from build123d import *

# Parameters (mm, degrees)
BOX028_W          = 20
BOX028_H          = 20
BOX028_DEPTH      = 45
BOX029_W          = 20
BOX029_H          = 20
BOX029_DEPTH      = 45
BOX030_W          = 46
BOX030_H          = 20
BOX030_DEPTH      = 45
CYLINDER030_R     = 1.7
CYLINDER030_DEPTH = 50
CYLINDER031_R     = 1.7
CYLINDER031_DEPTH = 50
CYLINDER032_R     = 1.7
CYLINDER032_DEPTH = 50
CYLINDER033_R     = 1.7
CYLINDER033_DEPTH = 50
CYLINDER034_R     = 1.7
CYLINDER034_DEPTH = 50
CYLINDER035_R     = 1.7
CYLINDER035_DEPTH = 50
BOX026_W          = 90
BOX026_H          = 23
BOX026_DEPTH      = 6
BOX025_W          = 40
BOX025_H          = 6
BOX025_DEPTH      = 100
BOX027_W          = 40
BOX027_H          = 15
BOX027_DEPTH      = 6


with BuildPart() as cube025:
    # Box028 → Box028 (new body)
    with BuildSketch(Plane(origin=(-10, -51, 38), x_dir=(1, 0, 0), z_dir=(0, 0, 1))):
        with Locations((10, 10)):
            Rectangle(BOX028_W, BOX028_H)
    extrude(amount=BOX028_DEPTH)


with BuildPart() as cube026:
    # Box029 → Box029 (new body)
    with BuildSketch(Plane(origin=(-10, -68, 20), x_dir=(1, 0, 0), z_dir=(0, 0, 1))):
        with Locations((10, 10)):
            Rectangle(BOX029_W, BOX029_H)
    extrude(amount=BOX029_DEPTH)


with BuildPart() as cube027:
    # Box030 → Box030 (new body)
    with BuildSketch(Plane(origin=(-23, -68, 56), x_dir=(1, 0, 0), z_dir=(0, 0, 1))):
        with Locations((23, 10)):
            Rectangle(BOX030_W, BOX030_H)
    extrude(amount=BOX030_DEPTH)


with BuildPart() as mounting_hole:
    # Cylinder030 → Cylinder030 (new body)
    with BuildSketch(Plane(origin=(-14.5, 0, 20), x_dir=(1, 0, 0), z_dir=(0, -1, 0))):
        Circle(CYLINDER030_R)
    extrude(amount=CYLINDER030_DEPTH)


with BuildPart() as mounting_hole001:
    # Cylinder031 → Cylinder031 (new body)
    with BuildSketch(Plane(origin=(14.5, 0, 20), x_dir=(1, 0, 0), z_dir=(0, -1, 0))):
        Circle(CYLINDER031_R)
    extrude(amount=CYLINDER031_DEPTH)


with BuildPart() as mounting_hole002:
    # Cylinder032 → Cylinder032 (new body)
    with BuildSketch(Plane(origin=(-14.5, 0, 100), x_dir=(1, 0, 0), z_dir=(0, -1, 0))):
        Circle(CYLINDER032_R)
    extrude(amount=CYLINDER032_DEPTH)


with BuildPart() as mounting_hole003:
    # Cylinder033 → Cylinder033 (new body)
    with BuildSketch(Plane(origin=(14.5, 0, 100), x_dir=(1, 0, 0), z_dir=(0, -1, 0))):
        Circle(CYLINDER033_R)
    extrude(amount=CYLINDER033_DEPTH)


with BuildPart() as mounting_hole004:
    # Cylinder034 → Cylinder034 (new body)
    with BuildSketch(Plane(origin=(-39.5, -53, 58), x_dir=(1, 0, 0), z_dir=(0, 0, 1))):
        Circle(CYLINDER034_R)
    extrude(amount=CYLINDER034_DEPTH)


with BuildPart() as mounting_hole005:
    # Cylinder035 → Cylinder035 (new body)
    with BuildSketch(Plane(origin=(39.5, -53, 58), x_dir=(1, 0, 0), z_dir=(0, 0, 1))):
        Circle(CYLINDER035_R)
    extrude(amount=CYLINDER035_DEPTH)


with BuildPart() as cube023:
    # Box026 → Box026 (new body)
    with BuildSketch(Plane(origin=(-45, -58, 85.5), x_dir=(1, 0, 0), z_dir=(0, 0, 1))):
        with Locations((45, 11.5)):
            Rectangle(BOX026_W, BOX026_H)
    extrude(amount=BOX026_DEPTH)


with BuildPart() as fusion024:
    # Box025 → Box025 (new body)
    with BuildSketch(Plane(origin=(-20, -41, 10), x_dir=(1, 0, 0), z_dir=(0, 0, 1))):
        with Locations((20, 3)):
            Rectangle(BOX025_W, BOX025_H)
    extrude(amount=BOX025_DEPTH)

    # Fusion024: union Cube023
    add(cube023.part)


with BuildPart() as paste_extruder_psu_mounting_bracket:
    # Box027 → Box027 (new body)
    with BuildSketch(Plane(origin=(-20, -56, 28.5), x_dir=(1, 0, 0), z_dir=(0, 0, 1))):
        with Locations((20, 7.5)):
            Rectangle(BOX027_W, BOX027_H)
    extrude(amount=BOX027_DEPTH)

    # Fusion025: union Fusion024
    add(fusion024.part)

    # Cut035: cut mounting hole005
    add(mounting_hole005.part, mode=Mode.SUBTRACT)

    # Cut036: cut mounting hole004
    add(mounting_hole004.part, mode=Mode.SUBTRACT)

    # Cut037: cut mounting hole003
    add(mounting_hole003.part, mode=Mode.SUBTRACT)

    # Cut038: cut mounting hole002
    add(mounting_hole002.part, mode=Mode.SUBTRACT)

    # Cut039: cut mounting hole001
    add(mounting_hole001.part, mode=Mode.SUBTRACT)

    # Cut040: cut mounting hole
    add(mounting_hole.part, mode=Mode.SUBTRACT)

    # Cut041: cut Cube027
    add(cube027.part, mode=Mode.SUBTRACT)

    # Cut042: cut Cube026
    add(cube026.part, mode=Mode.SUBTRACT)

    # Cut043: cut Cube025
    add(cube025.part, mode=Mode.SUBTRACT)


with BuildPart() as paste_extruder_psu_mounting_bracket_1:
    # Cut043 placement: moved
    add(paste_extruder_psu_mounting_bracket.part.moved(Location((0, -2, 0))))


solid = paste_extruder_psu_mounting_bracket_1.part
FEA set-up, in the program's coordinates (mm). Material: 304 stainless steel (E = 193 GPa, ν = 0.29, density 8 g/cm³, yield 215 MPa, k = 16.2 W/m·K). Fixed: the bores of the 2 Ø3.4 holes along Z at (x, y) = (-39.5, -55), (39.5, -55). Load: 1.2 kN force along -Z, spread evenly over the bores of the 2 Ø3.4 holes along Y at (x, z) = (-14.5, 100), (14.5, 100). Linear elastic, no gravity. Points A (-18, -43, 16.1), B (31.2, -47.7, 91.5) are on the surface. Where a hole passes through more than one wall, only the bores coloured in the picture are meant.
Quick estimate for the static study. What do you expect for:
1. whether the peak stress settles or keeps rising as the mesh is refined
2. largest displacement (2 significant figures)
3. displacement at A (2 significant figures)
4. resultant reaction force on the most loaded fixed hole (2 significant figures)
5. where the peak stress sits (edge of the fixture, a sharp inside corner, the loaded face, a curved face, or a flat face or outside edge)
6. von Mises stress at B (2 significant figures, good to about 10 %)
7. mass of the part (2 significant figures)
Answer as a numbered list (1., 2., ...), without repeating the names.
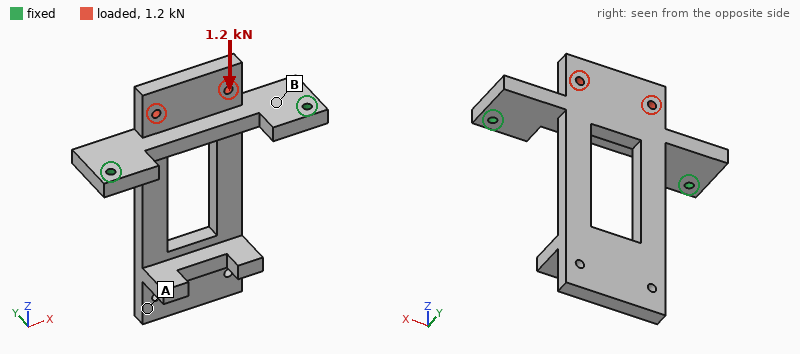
1. keeps rising
2. 0.15 mm
3. 0.13 mm
4. 600 N
5. edge of the fixture
6. 40 MPa
7. 230 g
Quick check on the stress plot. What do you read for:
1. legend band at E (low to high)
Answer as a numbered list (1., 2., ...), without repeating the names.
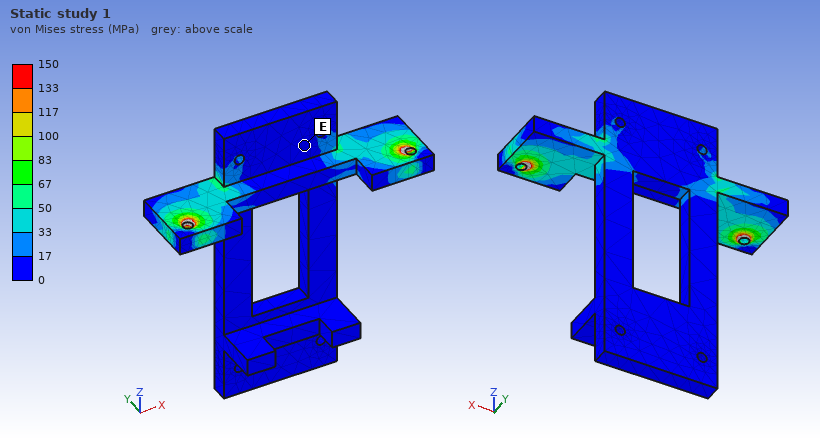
1. 0 to 17 MPa
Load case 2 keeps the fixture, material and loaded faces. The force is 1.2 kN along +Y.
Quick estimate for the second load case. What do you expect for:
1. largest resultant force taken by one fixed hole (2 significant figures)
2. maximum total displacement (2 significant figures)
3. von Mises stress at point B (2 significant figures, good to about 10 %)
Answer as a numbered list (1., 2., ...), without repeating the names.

1. 1.0 kN
2. 0.22 mm
3. 64 MPa
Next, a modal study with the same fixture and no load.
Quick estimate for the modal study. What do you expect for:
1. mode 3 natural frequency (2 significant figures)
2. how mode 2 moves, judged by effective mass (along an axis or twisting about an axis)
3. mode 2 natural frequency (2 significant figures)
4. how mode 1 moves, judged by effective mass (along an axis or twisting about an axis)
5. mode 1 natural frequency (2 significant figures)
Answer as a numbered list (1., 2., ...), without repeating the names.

1. 1900 Hz
2. along X
3. 1300 Hz
4. along Y
5. 400 Hz
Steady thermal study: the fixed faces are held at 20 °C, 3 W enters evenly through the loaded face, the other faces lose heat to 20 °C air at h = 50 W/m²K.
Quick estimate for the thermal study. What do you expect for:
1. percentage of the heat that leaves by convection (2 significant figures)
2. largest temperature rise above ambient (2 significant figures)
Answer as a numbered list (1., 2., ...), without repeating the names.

1. 79 %
2. 16 K
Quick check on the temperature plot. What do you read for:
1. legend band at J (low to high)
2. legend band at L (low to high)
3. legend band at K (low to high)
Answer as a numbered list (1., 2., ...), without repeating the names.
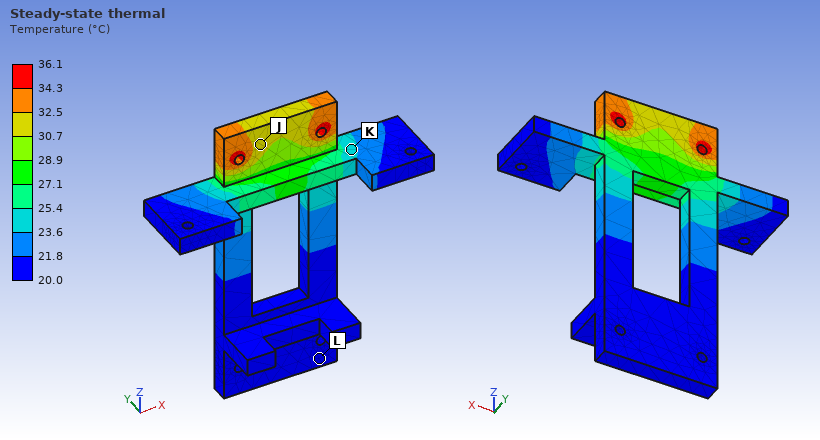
1. 30.7 to 32.5 °C
2. 20.0 to 21.8 °C
3. 23.6 to 25.4 °C
